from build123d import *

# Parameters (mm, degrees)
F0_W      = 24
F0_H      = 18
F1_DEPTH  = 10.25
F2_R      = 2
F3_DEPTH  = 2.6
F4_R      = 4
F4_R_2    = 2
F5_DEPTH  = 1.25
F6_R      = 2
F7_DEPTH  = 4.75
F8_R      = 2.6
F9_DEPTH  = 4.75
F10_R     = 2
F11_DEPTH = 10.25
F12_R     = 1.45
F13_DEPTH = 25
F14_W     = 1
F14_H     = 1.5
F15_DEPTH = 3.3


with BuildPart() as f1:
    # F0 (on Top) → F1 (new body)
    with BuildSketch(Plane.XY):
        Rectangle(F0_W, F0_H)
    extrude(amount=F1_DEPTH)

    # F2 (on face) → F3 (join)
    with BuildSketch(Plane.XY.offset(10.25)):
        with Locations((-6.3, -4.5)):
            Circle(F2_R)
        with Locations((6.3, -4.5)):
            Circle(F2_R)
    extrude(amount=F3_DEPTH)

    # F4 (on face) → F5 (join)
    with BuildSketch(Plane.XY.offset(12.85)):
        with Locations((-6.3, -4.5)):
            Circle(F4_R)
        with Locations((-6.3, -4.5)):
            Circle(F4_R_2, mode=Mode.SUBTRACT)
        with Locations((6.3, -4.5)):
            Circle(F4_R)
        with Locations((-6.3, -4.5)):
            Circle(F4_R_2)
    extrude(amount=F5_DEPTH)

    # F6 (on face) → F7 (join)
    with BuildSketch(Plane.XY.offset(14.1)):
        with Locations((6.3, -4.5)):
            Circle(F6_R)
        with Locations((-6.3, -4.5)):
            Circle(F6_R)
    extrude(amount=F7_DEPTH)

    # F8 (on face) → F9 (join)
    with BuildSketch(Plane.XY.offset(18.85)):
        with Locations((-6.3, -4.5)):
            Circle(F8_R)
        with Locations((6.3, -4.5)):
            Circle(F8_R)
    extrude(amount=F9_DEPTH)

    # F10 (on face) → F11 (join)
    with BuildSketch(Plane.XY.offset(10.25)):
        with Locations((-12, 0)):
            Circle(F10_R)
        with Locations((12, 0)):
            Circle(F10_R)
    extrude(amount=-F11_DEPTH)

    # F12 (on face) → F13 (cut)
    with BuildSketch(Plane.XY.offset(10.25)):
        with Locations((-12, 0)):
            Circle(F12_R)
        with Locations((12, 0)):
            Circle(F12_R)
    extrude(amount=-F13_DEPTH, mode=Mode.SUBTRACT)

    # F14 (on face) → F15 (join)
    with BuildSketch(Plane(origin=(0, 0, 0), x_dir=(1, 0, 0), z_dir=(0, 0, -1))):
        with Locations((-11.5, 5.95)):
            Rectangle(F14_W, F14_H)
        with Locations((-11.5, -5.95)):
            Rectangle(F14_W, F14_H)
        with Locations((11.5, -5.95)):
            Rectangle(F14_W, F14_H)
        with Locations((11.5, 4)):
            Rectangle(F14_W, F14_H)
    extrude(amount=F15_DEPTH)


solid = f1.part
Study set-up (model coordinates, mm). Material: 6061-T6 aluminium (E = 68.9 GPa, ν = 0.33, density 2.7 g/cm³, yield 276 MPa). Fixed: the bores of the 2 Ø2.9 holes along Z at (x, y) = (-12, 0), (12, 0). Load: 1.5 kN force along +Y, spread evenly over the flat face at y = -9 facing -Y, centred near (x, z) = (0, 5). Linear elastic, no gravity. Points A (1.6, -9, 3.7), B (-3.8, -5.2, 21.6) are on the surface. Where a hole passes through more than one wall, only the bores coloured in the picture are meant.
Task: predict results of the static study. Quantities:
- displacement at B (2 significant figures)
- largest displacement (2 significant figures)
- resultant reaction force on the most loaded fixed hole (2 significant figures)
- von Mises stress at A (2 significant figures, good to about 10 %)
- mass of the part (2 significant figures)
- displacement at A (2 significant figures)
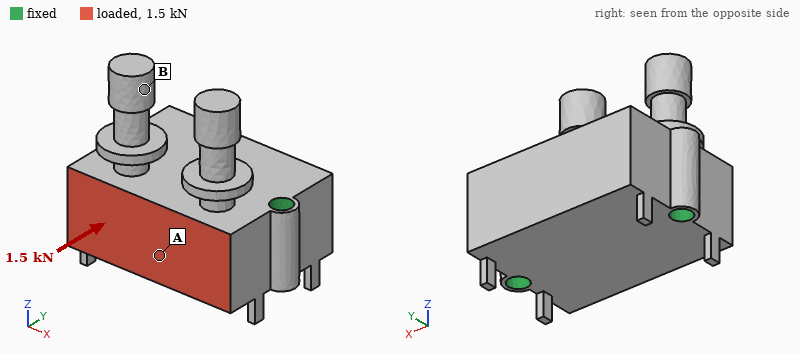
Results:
1.9 µm
2.2 µm
760 N
7.1 MPa
13 g
2.1 µm
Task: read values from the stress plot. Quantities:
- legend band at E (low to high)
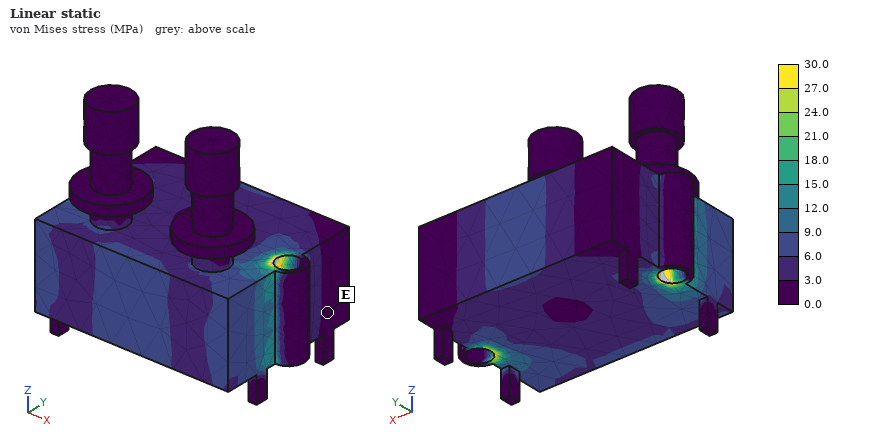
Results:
0.0 to 3.0 MPa
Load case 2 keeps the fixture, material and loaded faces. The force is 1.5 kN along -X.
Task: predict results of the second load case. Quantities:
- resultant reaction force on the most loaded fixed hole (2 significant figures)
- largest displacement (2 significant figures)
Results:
940 N
3.9 µm
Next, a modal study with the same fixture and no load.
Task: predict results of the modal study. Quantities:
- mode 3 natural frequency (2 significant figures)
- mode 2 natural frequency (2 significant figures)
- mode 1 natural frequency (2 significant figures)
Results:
11 kHz
11 kHz
11 kHz
